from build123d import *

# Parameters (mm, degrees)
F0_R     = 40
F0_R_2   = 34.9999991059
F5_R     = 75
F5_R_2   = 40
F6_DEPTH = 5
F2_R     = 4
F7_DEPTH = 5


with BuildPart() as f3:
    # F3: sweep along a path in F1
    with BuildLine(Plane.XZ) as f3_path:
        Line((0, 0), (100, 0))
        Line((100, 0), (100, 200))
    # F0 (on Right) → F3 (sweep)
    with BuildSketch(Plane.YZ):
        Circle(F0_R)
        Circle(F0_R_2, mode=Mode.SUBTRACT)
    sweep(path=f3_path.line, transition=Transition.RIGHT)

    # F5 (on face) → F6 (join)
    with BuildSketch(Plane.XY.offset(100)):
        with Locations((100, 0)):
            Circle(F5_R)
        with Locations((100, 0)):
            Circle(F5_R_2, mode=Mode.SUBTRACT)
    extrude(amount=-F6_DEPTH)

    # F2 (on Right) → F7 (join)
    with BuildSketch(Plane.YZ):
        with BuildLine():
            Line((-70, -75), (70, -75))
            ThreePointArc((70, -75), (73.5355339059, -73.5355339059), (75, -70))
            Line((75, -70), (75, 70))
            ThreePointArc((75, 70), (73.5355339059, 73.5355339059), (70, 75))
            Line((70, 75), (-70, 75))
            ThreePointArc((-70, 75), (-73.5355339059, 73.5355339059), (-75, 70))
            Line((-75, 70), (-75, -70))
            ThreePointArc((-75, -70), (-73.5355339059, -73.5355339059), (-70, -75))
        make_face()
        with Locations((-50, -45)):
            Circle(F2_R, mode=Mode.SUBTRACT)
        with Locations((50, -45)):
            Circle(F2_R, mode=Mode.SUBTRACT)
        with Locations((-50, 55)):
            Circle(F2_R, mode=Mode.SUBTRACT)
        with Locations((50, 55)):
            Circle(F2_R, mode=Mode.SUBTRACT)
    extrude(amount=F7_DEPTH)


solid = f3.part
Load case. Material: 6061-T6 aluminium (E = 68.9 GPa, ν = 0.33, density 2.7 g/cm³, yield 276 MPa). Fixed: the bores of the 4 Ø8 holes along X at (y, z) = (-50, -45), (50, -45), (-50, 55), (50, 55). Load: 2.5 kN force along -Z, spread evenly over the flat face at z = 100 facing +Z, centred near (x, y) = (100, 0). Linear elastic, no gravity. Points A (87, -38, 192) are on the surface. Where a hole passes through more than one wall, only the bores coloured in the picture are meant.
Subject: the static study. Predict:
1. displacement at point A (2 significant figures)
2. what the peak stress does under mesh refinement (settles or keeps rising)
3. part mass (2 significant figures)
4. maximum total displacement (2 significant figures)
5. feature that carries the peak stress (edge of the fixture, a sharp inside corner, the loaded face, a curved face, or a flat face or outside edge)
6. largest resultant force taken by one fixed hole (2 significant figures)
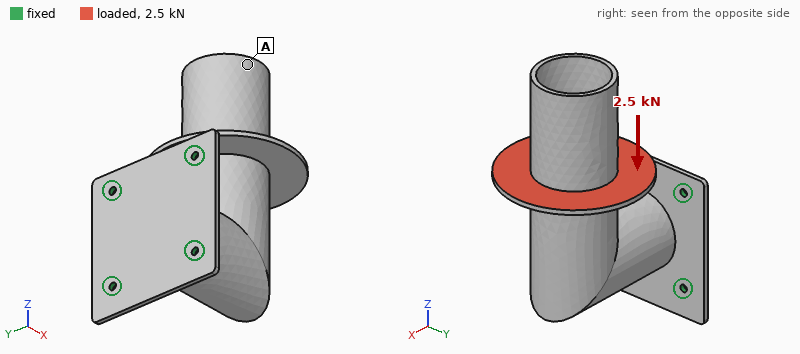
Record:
0.90 mm
keeps rising
1.4 kg
1.0 mm
edge of the fixture
1.6 kN
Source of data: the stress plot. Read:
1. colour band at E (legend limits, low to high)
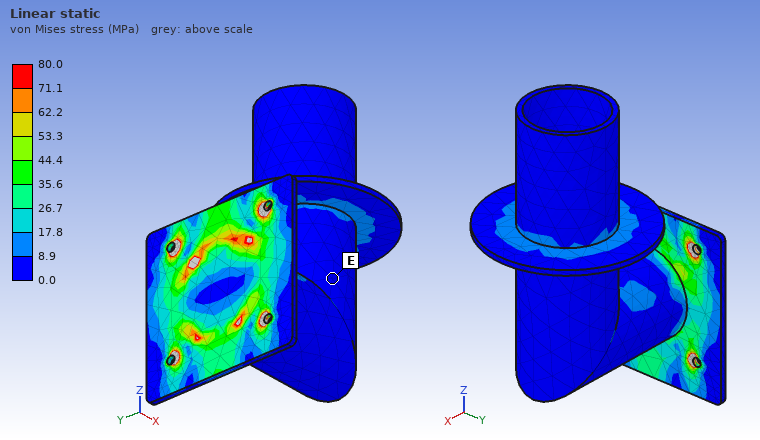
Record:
0.0 to 8.9 MPa
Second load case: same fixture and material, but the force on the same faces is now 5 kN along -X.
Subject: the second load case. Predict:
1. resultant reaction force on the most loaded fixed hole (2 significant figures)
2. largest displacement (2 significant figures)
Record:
4.1 kN
2.8 mm
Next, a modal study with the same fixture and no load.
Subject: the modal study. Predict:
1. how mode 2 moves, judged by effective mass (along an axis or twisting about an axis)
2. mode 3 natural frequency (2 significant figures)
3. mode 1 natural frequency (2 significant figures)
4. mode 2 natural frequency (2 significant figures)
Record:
along Y
900 Hz
250 Hz
330 Hz
